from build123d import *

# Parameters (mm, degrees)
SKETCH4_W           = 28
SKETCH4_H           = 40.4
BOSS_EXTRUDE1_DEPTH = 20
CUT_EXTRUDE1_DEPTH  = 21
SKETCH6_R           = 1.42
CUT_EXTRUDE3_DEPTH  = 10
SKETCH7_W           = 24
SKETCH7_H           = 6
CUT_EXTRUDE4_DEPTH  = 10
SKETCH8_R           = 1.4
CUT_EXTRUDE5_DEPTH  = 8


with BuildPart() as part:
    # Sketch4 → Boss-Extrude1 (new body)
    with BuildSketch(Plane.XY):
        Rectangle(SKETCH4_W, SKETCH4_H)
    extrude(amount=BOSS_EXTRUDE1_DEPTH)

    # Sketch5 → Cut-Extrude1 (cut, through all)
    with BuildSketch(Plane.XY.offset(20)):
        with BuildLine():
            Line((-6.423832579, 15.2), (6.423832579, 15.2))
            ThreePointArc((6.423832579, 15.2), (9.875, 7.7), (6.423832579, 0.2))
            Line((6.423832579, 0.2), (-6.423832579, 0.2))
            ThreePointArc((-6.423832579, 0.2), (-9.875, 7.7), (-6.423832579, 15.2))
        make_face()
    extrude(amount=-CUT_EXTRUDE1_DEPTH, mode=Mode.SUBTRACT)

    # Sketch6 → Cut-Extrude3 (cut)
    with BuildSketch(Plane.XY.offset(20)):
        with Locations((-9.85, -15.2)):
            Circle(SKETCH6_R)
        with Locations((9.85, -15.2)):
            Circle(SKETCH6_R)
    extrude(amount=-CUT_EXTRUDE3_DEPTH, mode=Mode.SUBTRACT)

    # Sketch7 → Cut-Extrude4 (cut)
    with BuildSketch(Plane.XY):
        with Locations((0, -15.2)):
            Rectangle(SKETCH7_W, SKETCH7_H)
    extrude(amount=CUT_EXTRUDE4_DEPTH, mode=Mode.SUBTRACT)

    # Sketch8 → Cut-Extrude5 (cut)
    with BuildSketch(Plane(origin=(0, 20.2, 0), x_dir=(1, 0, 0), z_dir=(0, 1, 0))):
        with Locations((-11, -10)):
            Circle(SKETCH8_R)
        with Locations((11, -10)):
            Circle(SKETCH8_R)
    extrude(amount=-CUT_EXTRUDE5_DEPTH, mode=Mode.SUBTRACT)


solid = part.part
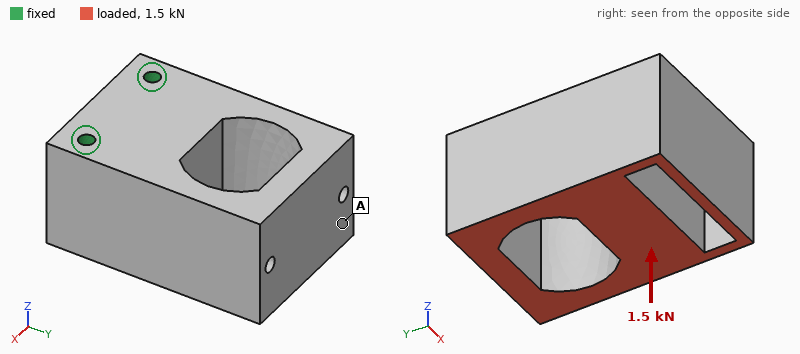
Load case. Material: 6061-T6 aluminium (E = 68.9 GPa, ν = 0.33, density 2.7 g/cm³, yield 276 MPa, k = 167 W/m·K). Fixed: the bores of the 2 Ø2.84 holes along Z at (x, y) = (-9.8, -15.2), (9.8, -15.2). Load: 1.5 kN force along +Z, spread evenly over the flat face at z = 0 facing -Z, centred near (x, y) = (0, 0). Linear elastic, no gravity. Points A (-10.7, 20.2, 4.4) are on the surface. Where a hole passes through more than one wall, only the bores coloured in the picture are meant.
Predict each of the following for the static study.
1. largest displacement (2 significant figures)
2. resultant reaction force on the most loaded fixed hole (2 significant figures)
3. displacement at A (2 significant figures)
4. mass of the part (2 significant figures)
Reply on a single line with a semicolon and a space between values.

45 µm; 750 N; 43 µm; 42 g
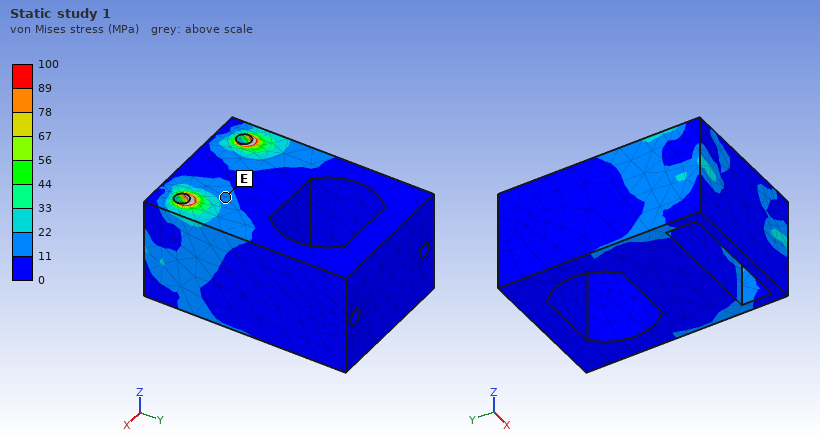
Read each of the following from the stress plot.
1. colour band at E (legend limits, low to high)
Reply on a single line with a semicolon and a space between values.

11 to 22 MPa
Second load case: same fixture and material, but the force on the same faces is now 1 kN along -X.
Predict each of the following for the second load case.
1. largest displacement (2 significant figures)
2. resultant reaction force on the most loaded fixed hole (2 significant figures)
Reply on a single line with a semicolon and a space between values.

17 µm; 1.1 kN
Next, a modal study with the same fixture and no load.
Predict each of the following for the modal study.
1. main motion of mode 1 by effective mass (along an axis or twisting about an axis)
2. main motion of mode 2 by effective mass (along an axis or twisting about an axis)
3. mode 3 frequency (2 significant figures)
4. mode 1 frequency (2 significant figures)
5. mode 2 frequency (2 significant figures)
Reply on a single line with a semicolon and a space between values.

along Z; along X; 13 kHz; 5600 Hz; 8500 Hz
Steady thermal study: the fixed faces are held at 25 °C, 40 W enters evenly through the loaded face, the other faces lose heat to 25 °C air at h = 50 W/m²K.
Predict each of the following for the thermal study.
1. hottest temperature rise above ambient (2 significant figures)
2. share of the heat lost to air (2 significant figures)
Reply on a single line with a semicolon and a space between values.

17 K; 6.2 %
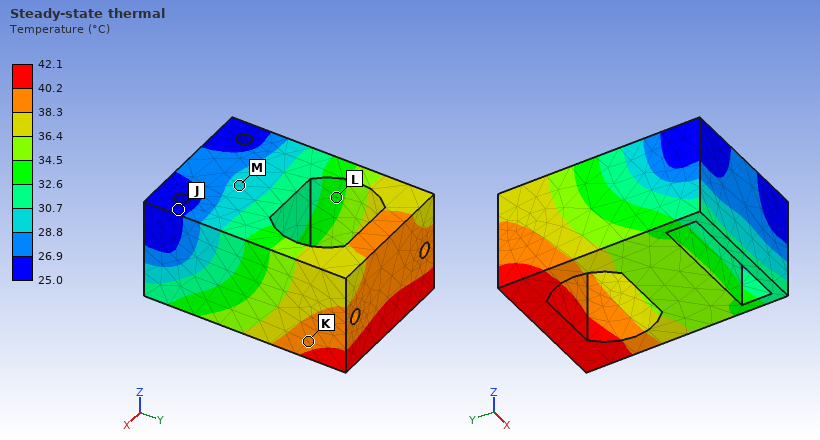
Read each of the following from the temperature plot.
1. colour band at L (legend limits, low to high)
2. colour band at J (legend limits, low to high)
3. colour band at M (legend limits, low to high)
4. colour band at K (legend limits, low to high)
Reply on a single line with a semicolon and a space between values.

32.6 to 34.5 °C; 25.0 to 26.9 °C; 28.8 to 30.7 °C; 38.3 to 40.2 °C
